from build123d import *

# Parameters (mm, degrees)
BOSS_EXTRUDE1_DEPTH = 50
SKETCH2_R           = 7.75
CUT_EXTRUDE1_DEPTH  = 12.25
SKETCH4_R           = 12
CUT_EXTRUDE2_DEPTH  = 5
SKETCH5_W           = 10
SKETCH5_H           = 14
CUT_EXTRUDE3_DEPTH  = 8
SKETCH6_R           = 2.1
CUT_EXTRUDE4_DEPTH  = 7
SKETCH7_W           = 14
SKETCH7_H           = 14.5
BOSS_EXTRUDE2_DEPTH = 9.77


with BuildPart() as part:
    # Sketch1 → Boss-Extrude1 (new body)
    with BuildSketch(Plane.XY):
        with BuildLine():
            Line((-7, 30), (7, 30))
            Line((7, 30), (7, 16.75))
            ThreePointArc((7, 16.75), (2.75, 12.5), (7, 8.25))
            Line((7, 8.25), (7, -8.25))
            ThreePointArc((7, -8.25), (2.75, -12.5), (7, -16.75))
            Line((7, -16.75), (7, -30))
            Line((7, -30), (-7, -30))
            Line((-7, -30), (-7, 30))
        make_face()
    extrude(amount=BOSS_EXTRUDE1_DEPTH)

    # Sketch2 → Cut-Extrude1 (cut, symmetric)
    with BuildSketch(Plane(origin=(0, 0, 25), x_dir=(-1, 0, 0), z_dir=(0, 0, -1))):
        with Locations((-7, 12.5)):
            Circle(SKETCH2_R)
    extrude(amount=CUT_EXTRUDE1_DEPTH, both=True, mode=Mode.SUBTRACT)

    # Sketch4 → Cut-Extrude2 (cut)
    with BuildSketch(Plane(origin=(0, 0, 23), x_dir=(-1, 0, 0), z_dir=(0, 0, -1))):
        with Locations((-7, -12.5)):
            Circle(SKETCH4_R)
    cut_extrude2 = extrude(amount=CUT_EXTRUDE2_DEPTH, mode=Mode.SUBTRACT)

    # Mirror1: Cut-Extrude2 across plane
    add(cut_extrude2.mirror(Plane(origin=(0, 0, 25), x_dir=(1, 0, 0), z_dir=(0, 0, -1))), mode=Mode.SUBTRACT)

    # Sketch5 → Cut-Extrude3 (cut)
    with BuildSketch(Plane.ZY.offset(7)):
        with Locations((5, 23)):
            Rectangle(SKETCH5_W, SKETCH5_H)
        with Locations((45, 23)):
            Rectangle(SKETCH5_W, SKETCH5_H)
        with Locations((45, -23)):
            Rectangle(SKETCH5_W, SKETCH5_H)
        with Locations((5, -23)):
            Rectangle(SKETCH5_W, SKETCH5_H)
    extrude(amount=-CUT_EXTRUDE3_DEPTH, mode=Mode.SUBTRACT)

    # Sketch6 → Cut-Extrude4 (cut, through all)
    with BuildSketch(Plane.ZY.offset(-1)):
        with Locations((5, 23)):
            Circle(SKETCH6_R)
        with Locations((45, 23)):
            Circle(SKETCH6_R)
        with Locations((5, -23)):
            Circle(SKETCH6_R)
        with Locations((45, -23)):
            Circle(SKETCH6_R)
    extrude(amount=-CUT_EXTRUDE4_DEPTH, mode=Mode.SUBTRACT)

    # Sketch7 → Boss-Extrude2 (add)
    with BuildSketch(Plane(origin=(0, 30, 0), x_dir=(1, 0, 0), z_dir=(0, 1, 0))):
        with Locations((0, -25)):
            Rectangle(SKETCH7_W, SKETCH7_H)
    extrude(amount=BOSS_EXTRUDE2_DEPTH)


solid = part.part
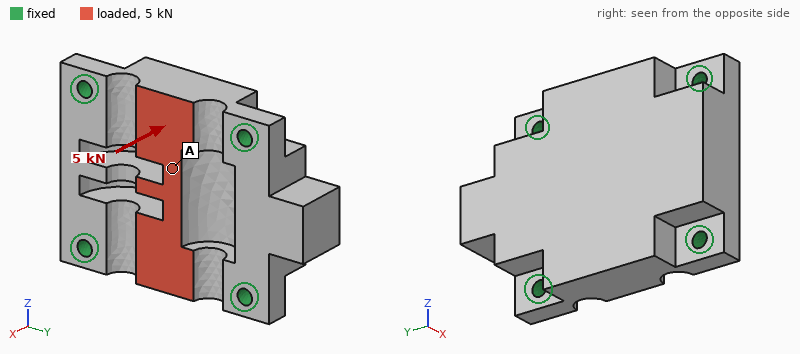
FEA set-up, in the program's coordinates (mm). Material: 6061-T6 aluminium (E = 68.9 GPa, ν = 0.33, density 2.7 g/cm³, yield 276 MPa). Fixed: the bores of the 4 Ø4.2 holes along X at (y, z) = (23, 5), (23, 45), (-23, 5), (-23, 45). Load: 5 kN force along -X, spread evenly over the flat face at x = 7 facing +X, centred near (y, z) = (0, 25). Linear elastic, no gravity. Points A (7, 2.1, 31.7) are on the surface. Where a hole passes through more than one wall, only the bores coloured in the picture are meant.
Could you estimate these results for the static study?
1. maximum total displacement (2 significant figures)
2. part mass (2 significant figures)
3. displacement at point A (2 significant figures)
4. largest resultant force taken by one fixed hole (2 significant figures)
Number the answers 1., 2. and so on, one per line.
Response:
1. 17 µm
2. 88 g
3. 16 µm
4. 1.7 kN
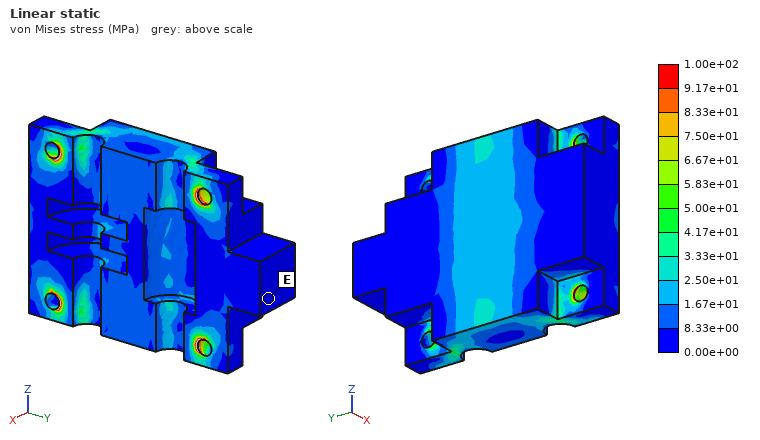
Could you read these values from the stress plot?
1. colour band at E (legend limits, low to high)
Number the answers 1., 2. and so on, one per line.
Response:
1. 0.00e+00 to 8.33e+00 MPa
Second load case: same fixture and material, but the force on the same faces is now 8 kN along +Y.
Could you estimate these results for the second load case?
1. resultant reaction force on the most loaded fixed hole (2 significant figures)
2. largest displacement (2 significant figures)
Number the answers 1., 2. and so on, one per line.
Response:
1. 2.2 kN
2. 22 µm
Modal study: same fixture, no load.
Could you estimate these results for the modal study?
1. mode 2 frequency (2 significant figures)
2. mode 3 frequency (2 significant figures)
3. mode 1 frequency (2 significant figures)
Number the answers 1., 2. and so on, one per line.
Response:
1. 14 kHz
2. 17 kHz
3. 13 kHz
